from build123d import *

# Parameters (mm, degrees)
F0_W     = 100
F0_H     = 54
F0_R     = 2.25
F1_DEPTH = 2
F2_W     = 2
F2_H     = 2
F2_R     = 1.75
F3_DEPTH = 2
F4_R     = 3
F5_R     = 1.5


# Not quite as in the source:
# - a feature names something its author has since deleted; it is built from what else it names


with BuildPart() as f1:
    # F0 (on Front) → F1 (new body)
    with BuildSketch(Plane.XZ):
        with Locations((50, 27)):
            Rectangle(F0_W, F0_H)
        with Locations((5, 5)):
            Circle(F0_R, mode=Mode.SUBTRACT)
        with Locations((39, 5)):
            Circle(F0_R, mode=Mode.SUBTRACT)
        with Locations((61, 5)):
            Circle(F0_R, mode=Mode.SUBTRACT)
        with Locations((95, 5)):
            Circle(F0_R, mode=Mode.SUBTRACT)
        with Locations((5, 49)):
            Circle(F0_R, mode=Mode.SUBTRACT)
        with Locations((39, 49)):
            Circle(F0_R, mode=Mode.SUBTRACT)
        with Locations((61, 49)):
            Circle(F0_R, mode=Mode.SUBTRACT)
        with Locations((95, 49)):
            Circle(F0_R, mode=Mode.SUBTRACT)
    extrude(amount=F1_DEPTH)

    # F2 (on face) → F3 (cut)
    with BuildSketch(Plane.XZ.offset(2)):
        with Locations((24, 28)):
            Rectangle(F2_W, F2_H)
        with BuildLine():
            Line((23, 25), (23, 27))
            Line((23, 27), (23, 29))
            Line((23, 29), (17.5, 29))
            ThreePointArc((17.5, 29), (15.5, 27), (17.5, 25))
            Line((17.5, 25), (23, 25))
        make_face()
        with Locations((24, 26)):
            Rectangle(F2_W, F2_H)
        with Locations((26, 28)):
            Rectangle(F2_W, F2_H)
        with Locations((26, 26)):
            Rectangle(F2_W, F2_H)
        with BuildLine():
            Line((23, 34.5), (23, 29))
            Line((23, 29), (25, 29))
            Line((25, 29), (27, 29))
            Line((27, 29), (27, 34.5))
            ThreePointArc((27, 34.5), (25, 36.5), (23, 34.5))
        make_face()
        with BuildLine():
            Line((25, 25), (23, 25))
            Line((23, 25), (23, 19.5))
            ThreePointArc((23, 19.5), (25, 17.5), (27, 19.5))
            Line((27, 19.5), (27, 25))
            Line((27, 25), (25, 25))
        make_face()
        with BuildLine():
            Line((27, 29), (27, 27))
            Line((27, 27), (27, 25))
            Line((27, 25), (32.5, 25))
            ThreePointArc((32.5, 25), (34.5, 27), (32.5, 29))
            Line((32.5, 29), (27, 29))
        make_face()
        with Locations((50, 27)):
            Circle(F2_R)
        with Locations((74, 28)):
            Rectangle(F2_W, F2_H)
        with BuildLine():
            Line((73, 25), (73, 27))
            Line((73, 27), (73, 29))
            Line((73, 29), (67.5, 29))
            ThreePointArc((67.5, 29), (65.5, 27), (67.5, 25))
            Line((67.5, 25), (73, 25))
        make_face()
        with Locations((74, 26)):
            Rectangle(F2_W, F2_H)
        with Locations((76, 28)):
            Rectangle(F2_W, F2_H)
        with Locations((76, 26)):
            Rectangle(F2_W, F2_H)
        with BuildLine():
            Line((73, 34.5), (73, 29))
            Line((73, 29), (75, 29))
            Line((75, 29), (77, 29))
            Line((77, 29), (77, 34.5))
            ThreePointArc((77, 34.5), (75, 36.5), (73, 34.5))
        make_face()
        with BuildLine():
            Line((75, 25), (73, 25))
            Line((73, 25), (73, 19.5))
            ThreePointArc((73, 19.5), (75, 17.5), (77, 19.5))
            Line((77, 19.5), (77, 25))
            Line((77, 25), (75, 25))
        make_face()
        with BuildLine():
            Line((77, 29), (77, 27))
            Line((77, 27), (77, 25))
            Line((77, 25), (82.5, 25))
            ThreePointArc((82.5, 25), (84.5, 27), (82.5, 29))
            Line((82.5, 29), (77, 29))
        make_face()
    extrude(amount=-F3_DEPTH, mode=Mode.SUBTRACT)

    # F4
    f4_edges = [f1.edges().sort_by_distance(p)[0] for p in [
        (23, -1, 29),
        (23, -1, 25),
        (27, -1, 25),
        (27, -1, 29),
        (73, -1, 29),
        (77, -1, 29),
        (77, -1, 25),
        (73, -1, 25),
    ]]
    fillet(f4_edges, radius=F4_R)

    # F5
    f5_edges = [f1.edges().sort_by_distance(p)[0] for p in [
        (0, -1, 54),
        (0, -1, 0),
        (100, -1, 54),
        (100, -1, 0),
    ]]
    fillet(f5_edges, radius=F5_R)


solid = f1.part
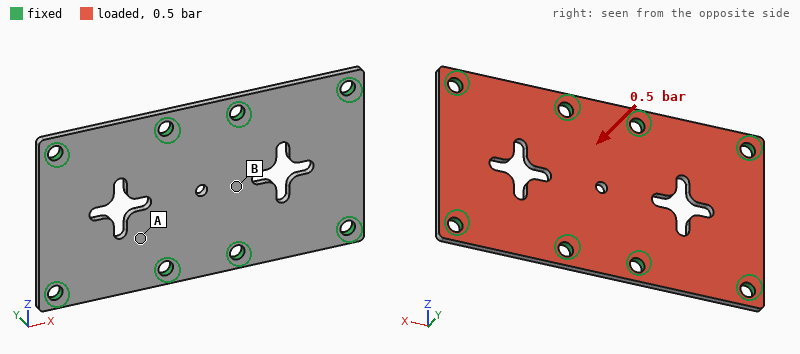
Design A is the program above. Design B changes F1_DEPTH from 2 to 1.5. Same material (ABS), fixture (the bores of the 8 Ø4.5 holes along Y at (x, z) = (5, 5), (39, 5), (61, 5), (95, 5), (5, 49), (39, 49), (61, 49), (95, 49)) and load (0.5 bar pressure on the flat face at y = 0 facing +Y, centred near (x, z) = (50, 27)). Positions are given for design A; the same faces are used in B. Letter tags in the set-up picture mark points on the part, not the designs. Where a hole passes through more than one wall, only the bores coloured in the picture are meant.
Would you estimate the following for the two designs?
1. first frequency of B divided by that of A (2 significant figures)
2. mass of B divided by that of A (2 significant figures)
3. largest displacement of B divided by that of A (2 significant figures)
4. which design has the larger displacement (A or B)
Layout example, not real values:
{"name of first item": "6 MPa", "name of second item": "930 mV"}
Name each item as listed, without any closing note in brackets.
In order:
{"first frequency of B divided by that of A": "0.76", "mass of B divided by that of A": "0.75", "largest displacement of B divided by that of A": "2.3", "which design has the larger displacement": "B"}
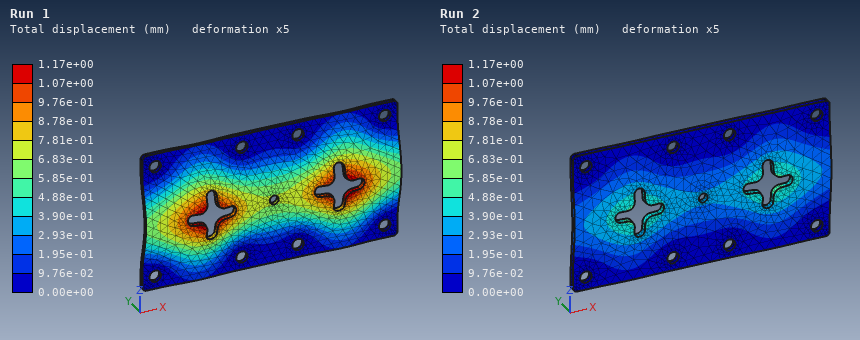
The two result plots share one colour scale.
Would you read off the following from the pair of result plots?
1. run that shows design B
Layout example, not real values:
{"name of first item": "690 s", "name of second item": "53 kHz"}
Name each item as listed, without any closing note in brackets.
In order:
{"run that shows design B": "Run 1"}
